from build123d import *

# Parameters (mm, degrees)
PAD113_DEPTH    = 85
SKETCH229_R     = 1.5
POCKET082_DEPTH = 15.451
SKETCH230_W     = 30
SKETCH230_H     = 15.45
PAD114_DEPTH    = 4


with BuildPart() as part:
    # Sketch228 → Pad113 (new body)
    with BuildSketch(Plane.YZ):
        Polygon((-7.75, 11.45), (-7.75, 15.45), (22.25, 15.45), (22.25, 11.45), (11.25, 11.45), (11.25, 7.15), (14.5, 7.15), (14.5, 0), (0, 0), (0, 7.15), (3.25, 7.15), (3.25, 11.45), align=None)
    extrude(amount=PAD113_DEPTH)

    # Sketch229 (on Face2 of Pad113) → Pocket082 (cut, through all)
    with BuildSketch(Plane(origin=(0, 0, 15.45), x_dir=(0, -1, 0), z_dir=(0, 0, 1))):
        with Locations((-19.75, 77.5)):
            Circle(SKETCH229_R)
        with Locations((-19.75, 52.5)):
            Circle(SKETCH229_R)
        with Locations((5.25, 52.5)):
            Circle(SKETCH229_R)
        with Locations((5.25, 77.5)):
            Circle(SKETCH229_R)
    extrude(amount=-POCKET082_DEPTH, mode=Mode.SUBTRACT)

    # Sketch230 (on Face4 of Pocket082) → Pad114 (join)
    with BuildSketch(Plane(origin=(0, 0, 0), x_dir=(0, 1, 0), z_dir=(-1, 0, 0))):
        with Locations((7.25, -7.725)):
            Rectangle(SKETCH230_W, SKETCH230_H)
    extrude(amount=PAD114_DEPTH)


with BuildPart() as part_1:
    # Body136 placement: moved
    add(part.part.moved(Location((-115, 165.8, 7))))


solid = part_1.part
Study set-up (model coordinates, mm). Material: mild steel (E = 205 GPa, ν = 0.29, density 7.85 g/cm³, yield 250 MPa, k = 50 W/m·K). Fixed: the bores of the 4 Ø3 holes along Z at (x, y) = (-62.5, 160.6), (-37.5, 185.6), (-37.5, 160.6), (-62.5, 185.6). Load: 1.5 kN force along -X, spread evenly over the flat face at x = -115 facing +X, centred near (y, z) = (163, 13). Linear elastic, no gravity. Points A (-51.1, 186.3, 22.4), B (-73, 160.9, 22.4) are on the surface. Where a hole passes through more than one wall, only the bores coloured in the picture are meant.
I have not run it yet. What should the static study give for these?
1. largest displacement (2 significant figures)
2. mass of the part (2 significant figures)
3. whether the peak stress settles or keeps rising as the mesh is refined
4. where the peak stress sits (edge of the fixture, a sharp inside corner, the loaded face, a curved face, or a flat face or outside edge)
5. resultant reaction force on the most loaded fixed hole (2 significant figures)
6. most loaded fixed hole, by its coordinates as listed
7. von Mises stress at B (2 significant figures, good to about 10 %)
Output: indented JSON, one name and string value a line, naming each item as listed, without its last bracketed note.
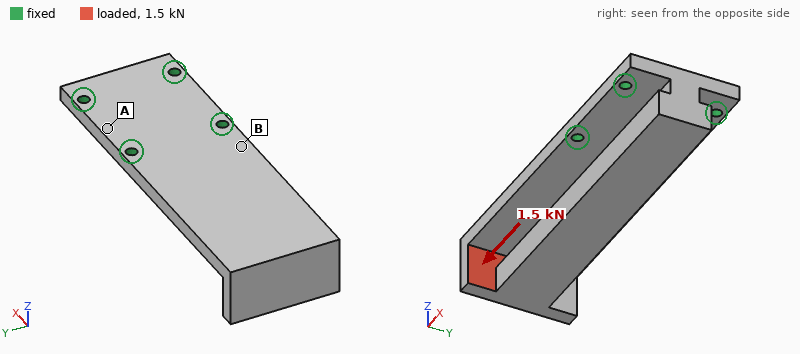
{
  "largest displacement": "34 µm",
  "mass of the part": "190 g",
  "whether the peak stress settles or keeps rising as the mesh is refined": "keeps rising",
  "where the peak stress sits": "edge of the fixture",
  "resultant reaction force on the most loaded fixed hole": "1.0 kN",
  "most loaded fixed hole, by its coordinates as listed": "(-62.5, 160.6)",
  "von Mises stress at B": "21 MPa"
}
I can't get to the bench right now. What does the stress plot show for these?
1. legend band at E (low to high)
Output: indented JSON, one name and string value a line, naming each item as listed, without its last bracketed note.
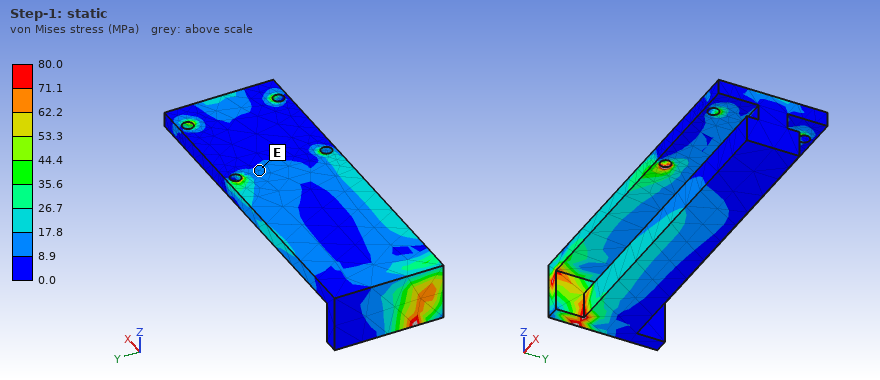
{
  "legend band at E": "8.9 to 17.8 MPa"
}
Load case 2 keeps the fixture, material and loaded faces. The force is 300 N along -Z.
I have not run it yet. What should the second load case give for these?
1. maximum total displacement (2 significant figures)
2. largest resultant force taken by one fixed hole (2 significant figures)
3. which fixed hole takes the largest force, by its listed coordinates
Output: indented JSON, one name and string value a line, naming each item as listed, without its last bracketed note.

{
  "maximum total displacement": "45 µm",
  "largest resultant force taken by one fixed hole": "590 N",
  "which fixed hole takes the largest force, by its listed coordinates": "(-62.5, 160.6)"
}
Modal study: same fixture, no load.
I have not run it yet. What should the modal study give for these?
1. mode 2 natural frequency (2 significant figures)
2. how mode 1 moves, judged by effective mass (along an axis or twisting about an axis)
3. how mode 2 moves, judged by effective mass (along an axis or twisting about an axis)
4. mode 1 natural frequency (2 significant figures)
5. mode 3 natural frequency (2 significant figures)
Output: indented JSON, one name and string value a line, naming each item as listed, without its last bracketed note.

{
  "mode 2 natural frequency": "4000 Hz",
  "how mode 1 moves, judged by effective mass": "along Z",
  "how mode 2 moves, judged by effective mass": "along Y",
  "mode 1 natural frequency": "2100 Hz",
  "mode 3 natural frequency": "6200 Hz"
}
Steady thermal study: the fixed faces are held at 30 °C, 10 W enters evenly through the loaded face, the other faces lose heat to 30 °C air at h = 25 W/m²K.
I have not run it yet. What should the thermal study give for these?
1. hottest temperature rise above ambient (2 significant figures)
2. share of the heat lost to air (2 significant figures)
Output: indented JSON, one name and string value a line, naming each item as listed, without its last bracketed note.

{
  "hottest temperature rise above ambient": "58 K",
  "share of the heat lost to air": "37 %"
}
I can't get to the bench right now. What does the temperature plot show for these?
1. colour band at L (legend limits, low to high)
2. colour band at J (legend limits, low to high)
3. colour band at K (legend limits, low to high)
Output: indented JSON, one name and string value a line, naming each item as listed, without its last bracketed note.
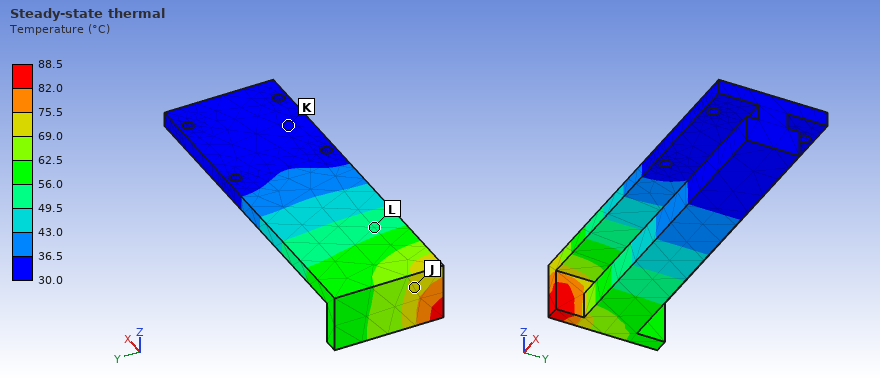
{
  "colour band at L": "49.5 to 56.0 °C",
  "colour band at J": "69.0 to 75.5 °C",
  "colour band at K": "30.0 to 36.5 °C"
}
